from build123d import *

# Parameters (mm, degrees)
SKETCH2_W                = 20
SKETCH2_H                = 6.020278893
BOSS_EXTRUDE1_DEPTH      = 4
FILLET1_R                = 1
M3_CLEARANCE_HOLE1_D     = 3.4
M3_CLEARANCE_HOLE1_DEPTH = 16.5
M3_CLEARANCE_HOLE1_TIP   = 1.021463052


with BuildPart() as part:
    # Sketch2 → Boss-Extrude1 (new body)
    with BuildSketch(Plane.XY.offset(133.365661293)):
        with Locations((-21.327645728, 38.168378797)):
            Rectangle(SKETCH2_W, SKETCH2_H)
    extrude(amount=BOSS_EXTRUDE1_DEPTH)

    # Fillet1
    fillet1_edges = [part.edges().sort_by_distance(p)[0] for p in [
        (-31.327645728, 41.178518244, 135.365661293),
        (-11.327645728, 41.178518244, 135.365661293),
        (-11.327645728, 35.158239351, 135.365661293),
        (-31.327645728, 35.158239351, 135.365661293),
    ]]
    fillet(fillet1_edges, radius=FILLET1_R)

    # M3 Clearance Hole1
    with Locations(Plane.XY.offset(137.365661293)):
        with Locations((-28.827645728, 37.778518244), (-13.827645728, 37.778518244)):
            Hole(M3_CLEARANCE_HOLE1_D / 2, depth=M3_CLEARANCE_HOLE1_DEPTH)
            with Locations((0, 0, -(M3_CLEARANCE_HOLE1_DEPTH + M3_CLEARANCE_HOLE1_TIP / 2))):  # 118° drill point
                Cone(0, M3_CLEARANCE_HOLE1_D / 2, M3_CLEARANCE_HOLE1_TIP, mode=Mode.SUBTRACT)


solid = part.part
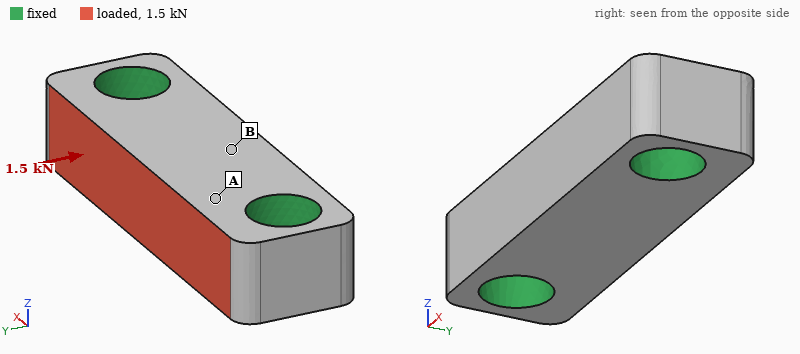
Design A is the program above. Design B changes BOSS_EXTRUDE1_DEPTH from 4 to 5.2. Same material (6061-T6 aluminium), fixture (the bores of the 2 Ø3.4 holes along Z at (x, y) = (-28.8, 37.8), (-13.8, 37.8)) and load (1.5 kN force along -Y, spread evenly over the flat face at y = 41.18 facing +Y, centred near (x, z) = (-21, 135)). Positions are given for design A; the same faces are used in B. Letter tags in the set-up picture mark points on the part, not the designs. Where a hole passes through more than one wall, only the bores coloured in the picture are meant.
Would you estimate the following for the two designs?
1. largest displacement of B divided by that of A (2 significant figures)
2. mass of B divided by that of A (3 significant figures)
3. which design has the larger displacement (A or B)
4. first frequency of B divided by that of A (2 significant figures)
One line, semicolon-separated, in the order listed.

0.78; 1.30; A; 1.1
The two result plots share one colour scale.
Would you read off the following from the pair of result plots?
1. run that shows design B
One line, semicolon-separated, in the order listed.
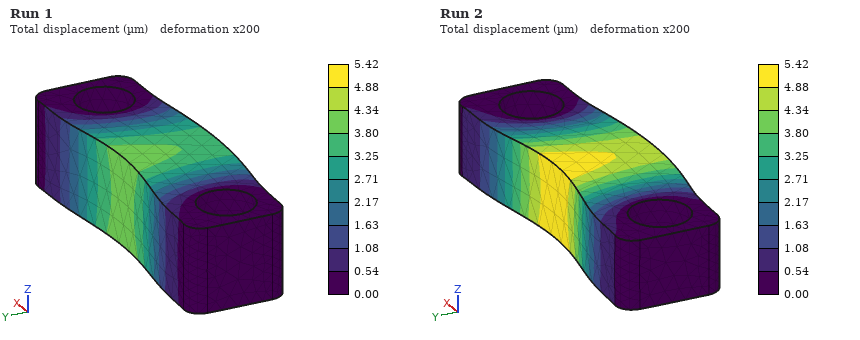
Run 1
